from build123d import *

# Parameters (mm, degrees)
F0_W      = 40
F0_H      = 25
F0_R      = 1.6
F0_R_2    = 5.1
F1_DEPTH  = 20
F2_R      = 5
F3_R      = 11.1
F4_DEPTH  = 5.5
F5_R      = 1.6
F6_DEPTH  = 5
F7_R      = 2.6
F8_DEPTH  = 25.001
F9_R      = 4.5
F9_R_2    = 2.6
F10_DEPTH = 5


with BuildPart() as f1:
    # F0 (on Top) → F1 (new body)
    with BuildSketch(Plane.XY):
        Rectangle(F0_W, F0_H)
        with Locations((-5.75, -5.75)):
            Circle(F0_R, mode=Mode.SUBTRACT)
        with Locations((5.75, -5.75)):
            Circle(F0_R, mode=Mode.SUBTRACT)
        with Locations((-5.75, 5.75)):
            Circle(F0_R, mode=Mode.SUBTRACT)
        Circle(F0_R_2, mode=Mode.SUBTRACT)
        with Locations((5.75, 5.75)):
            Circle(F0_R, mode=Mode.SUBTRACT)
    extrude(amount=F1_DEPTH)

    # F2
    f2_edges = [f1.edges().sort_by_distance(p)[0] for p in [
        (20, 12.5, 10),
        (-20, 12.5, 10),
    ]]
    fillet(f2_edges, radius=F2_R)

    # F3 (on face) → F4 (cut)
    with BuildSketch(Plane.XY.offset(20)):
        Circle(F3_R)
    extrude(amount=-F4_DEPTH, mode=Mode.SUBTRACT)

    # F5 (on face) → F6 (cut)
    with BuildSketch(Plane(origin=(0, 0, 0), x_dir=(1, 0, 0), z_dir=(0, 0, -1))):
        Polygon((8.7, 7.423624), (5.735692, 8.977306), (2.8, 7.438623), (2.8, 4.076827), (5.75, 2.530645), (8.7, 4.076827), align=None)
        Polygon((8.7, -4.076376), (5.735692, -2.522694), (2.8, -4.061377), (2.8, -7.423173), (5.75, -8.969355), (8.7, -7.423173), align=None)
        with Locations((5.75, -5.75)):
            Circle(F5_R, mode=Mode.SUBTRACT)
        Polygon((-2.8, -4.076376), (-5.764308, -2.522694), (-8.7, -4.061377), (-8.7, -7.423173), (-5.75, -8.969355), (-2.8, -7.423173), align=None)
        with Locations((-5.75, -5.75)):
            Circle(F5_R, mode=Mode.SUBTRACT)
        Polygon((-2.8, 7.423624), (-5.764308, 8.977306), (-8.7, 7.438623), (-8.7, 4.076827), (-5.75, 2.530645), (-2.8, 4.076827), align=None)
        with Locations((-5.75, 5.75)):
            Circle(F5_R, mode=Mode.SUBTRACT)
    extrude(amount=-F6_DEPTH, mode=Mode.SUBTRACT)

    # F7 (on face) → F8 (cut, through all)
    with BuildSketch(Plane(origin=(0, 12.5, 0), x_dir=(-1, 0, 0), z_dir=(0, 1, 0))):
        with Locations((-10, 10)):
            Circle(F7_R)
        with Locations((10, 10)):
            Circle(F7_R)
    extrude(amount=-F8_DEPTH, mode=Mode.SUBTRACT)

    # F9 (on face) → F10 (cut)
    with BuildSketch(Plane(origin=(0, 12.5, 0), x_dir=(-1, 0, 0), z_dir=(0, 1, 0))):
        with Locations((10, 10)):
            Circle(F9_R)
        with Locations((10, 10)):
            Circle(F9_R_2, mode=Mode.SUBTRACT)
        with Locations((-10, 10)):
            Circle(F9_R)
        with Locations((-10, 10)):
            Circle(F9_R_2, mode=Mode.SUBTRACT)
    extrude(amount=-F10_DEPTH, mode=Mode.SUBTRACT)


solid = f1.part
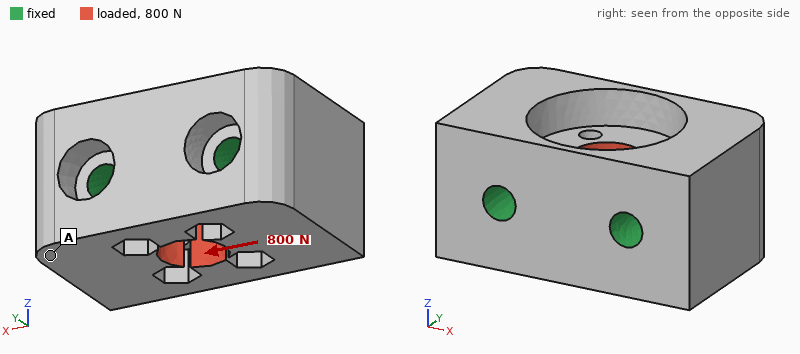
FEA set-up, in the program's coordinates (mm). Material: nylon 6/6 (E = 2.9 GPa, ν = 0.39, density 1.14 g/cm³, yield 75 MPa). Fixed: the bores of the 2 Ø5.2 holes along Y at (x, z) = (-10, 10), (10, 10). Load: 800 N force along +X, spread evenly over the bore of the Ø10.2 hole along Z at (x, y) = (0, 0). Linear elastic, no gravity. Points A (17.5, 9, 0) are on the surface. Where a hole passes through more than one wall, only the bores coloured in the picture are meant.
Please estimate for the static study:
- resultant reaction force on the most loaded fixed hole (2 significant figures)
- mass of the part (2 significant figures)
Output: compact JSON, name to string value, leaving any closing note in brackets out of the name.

{"resultant reaction force on the most loaded fixed hole": "410 N", "mass of the part": "16 g"}
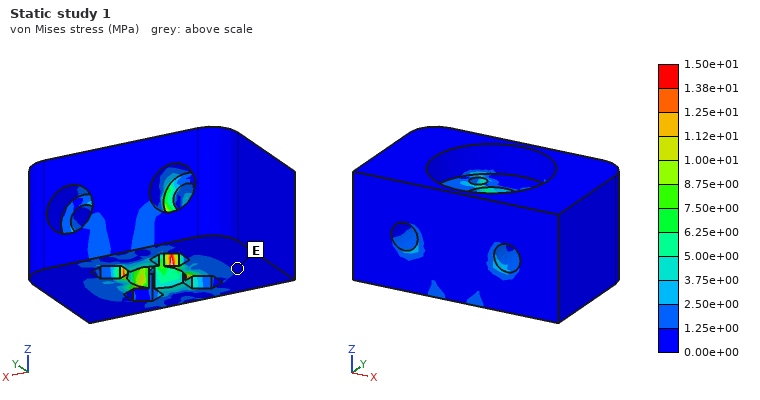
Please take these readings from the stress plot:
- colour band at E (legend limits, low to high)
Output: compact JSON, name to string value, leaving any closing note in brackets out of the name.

{"colour band at E": "0.00e+00 to 1.25e+00 MPa"}
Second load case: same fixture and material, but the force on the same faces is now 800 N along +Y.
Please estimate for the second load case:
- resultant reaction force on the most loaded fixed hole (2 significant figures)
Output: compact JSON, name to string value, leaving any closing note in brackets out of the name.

{"resultant reaction force on the most loaded fixed hole": "400 N"}
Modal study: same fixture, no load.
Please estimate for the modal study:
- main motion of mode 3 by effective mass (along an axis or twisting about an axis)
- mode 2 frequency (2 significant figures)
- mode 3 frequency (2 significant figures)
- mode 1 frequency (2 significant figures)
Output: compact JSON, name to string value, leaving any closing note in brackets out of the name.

{"main motion of mode 3 by effective mass": "along Z", "mode 2 frequency": "11 kHz", "mode 3 frequency": "12 kHz", "mode 1 frequency": "11 kHz"}
